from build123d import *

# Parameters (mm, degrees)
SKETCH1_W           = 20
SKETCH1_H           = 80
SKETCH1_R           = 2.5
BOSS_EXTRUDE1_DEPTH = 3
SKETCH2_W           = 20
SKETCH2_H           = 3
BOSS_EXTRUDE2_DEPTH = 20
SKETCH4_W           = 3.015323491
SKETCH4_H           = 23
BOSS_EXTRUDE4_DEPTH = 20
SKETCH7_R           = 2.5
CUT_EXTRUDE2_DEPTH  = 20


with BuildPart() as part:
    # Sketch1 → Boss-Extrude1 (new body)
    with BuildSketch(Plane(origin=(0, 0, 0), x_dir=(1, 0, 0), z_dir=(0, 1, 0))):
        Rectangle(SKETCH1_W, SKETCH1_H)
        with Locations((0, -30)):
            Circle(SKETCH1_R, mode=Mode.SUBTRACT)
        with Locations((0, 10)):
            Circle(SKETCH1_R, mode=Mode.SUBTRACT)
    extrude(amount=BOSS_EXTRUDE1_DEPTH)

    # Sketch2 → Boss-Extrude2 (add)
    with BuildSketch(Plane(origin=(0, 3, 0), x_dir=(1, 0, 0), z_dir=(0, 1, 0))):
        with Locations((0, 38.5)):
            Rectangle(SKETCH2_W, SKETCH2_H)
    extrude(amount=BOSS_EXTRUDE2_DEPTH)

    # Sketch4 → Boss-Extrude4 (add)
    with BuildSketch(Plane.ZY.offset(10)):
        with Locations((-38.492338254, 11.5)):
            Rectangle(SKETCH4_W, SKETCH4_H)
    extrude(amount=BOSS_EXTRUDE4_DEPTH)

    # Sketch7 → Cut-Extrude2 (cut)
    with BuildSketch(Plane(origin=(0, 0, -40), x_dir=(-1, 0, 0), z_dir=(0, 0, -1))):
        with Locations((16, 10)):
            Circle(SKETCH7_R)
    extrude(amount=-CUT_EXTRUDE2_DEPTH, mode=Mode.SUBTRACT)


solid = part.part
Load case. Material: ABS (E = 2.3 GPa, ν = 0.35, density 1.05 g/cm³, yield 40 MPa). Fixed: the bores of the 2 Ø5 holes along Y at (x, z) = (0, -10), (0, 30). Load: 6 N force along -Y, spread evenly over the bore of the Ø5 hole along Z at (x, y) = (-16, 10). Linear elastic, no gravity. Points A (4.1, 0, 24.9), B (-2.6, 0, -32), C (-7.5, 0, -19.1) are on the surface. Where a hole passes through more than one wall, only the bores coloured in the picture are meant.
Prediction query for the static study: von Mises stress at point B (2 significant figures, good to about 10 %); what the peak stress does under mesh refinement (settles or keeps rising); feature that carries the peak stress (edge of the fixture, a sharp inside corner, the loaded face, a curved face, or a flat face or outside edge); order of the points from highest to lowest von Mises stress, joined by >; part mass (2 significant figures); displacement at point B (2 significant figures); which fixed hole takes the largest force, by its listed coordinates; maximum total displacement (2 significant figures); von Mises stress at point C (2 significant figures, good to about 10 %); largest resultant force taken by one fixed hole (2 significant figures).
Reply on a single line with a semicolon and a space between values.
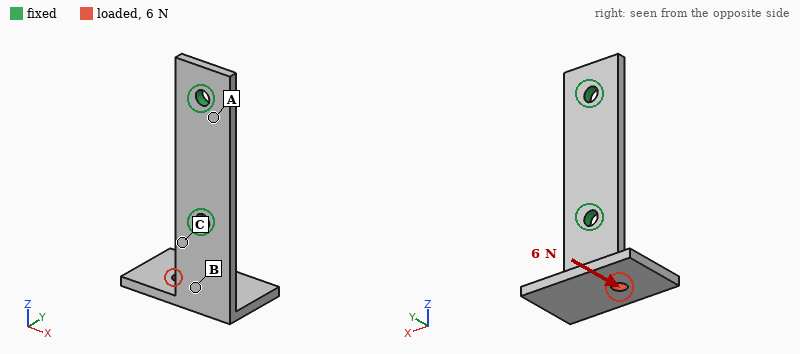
2.8 MPa; keeps rising; edge of the fixture; C > B > A; 7.6 g; 0.29 mm; (0, -10); 1.1 mm; 4.6 MPa; 6.2 N
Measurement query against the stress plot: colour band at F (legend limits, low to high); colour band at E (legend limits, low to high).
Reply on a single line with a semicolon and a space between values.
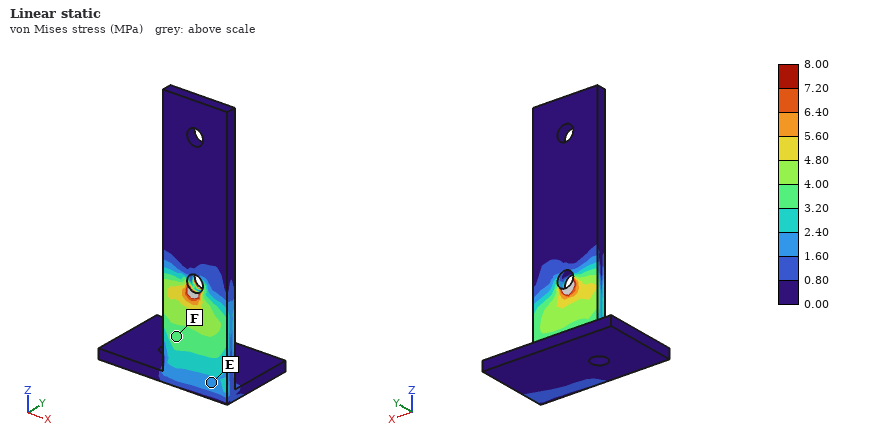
3.20 to 4.00 MPa; 1.60 to 2.40 MPa
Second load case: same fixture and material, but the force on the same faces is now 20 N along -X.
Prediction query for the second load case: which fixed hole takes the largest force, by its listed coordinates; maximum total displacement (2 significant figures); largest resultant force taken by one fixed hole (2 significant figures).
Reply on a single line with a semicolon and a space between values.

(0, -10); 1.1 mm; 29 N
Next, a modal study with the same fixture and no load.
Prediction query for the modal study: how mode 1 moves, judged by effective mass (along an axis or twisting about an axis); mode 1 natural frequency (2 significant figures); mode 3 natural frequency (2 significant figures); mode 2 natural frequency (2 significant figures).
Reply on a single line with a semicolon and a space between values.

along Y; 270 Hz; 790 Hz; 430 Hz
